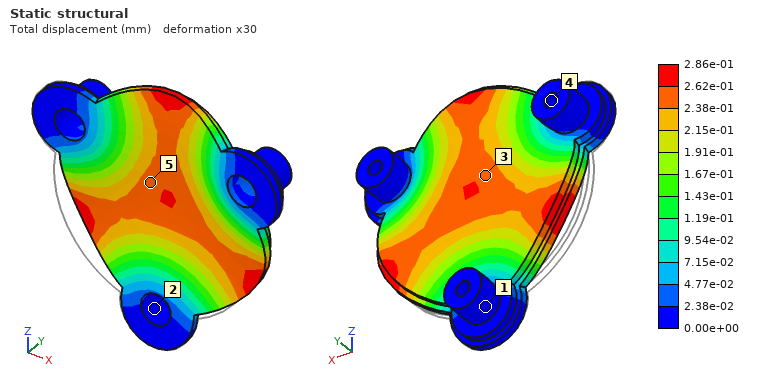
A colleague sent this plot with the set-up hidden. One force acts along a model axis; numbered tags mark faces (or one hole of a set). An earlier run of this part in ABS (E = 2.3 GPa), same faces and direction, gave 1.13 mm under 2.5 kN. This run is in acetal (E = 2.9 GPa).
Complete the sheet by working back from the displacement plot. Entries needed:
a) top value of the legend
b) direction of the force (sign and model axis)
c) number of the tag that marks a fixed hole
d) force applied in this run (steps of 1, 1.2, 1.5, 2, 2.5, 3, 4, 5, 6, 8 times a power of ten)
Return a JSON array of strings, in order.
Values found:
["2.86e-01 mm", "+Y", "4", "800 N"]
